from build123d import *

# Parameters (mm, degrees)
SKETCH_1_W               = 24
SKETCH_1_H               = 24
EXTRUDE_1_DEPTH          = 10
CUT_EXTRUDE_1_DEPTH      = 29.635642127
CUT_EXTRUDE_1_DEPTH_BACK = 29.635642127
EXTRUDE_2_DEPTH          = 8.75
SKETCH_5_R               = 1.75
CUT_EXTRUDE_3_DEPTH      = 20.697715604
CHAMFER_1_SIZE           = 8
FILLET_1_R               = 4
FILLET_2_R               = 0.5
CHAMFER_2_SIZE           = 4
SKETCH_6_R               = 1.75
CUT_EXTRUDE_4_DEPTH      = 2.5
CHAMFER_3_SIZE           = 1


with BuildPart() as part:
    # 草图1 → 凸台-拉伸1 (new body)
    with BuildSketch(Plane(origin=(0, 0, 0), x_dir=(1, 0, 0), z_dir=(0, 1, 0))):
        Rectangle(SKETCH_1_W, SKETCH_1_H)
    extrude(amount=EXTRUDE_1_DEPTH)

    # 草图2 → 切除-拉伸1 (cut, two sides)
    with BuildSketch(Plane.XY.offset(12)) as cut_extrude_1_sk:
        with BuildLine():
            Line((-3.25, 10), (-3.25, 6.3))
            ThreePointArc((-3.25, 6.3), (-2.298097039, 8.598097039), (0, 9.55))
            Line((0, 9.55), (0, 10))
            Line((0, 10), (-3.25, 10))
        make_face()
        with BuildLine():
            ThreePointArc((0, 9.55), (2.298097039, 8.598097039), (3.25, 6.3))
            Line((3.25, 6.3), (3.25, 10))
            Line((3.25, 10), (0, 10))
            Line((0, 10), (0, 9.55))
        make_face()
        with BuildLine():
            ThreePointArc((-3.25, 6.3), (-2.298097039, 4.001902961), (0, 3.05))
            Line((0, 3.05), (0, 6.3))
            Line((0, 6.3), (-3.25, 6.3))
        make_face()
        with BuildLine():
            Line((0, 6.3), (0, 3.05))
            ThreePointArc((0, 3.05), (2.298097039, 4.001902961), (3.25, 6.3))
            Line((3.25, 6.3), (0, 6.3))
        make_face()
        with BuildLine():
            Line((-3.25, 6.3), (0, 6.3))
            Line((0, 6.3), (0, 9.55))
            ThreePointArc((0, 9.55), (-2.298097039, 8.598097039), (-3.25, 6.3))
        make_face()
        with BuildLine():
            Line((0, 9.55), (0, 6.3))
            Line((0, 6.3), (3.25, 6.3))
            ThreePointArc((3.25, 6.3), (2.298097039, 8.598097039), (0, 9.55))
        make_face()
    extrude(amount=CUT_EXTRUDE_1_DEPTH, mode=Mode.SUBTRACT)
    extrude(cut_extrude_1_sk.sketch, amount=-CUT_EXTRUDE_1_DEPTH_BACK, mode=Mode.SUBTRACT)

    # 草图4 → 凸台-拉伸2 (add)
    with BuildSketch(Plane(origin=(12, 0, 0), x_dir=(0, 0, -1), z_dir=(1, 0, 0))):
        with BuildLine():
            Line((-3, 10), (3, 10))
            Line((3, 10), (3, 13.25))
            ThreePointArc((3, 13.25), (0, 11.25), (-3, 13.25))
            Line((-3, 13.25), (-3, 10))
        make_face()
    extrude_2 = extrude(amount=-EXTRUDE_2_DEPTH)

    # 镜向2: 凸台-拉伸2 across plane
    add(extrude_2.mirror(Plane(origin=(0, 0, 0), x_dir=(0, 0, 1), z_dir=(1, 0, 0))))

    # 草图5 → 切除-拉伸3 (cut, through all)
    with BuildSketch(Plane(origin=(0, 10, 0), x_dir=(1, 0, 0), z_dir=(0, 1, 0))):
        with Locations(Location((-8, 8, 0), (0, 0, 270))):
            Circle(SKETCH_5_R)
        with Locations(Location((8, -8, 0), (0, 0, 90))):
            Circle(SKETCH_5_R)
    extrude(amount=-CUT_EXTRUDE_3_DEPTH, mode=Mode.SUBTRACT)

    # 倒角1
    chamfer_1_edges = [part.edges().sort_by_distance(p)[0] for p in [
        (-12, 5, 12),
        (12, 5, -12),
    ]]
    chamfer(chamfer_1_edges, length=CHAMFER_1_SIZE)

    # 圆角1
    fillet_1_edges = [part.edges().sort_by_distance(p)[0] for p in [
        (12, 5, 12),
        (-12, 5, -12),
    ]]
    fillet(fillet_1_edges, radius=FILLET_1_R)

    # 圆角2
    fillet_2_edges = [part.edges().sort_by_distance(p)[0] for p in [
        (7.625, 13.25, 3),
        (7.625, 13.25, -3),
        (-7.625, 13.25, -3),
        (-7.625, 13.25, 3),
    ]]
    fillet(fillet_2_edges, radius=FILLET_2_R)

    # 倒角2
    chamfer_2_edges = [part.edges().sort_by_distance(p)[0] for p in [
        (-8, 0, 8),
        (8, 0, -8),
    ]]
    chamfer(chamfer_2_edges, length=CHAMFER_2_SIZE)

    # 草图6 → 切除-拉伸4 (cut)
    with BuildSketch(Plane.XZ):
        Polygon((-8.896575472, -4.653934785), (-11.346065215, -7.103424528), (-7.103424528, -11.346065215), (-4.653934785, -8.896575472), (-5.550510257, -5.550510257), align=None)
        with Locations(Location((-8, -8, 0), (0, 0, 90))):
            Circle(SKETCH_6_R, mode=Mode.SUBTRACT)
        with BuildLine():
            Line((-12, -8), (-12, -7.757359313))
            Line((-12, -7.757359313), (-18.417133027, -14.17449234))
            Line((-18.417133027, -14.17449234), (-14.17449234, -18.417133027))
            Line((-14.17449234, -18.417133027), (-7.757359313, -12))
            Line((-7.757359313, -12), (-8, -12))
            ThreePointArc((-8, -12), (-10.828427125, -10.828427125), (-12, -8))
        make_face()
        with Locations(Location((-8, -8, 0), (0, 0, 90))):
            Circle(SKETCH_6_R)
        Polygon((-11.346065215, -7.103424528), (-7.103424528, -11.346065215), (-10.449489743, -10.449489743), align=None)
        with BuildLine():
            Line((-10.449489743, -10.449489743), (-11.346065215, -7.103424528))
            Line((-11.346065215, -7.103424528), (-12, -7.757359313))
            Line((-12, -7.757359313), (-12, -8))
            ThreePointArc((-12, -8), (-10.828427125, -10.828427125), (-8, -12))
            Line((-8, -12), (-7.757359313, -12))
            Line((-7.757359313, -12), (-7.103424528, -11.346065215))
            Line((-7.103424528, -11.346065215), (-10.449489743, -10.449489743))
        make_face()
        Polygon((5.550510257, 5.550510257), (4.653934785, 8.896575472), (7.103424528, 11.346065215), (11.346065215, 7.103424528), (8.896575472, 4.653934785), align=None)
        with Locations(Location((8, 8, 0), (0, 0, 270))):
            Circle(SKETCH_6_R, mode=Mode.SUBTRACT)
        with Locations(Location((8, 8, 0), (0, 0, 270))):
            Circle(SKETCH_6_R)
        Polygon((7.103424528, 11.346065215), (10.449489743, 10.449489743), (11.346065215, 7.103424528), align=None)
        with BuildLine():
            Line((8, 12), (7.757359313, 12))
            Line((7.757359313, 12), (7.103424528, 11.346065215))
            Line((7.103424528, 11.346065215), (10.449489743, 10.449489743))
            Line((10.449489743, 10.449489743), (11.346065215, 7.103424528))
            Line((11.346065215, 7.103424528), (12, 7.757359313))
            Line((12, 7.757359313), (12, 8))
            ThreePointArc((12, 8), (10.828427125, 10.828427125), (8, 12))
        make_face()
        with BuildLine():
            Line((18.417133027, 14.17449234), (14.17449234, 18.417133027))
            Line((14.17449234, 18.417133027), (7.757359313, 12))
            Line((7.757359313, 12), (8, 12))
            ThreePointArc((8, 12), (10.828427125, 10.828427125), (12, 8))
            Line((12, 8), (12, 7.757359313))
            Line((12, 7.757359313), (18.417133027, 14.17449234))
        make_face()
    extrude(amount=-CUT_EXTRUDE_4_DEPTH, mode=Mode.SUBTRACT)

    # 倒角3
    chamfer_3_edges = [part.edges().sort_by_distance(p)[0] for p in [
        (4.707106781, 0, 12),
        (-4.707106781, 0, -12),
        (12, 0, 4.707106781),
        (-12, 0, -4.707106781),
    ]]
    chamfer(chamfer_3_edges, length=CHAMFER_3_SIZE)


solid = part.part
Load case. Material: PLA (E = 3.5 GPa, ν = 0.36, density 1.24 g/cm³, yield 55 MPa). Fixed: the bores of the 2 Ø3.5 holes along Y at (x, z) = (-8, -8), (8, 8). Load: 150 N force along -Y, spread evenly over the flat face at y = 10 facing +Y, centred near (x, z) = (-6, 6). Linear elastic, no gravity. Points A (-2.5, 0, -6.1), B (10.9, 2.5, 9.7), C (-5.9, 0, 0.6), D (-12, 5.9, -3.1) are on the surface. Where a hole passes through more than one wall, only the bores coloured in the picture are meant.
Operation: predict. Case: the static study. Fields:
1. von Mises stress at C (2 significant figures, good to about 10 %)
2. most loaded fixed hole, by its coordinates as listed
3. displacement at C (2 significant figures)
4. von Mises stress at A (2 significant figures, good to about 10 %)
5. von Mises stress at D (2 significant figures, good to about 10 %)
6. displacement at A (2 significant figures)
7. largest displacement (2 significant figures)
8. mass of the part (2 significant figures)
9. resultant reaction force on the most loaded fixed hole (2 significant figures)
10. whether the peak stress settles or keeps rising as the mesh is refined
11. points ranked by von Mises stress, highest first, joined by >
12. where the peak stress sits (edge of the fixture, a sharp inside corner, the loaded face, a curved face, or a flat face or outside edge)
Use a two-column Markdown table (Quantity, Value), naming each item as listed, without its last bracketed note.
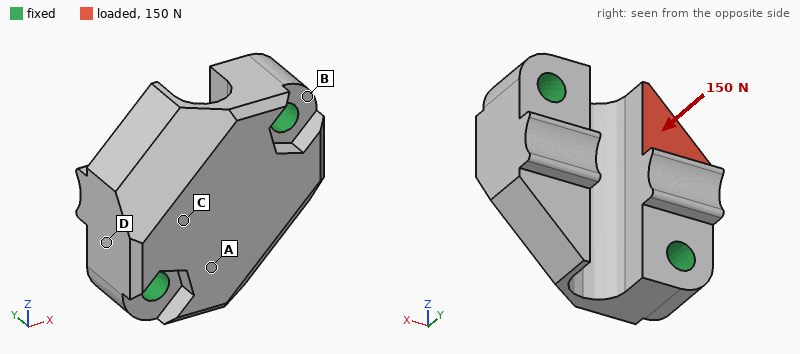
| Quantity | Value |
|---|---|
| von Mises stress at C | 4.2 MPa |
| most loaded fixed hole, by its coordinates as listed | (-8, -8) |
| displacement at C | 34 µm |
| von Mises stress at A | 2.5 MPa |
| von Mises stress at D | 6.6 MPa |
| displacement at A | 13 µm |
| largest displacement | 88 µm |
| mass of the part | 4.6 g |
| resultant reaction force on the most loaded fixed hole | 110 N |
| whether the peak stress settles or keeps rising as the mesh is refined | keeps rising |
| points ranked by von Mises stress, highest first, joined by > | D > C > A > B |
| where the peak stress sits | edge of the fixture |
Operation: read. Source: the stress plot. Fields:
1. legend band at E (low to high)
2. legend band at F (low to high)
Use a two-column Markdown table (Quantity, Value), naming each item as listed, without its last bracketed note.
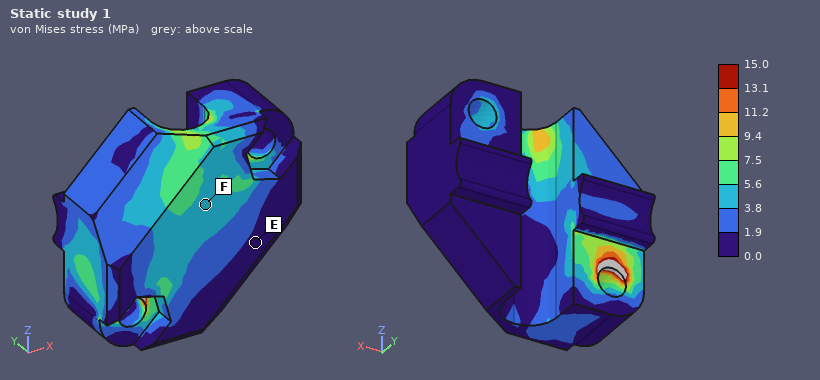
| Quantity | Value |
|---|---|
| legend band at E | 0.0 to 1.9 MPa |
| legend band at F | 3.8 to 5.6 MPa |
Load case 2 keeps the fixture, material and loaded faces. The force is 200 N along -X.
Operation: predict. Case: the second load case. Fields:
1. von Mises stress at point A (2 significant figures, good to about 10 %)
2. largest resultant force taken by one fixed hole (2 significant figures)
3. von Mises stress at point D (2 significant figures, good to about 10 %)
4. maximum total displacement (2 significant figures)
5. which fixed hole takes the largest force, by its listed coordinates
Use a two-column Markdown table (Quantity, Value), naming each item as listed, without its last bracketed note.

| Quantity | Value |
|---|---|
| von Mises stress at point A | 4.3 MPa |
| largest resultant force taken by one fixed hole | 140 N |
| von Mises stress at point D | 12 MPa |
| maximum total displacement | 0.16 mm |
| which fixed hole takes the largest force, by its listed coordinates | (-8, -8) |
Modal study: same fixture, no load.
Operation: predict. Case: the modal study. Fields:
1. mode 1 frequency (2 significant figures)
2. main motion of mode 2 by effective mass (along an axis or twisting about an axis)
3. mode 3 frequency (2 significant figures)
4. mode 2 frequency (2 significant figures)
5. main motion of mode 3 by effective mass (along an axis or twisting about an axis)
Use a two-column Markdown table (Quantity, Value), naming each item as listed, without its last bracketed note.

| Quantity | Value |
|---|---|
| mode 1 frequency | 8200 Hz |
| main motion of mode 2 by effective mass | along Y |
| mode 3 frequency | 11 kHz |
| mode 2 frequency | 9500 Hz |
| main motion of mode 3 by effective mass | along X |
